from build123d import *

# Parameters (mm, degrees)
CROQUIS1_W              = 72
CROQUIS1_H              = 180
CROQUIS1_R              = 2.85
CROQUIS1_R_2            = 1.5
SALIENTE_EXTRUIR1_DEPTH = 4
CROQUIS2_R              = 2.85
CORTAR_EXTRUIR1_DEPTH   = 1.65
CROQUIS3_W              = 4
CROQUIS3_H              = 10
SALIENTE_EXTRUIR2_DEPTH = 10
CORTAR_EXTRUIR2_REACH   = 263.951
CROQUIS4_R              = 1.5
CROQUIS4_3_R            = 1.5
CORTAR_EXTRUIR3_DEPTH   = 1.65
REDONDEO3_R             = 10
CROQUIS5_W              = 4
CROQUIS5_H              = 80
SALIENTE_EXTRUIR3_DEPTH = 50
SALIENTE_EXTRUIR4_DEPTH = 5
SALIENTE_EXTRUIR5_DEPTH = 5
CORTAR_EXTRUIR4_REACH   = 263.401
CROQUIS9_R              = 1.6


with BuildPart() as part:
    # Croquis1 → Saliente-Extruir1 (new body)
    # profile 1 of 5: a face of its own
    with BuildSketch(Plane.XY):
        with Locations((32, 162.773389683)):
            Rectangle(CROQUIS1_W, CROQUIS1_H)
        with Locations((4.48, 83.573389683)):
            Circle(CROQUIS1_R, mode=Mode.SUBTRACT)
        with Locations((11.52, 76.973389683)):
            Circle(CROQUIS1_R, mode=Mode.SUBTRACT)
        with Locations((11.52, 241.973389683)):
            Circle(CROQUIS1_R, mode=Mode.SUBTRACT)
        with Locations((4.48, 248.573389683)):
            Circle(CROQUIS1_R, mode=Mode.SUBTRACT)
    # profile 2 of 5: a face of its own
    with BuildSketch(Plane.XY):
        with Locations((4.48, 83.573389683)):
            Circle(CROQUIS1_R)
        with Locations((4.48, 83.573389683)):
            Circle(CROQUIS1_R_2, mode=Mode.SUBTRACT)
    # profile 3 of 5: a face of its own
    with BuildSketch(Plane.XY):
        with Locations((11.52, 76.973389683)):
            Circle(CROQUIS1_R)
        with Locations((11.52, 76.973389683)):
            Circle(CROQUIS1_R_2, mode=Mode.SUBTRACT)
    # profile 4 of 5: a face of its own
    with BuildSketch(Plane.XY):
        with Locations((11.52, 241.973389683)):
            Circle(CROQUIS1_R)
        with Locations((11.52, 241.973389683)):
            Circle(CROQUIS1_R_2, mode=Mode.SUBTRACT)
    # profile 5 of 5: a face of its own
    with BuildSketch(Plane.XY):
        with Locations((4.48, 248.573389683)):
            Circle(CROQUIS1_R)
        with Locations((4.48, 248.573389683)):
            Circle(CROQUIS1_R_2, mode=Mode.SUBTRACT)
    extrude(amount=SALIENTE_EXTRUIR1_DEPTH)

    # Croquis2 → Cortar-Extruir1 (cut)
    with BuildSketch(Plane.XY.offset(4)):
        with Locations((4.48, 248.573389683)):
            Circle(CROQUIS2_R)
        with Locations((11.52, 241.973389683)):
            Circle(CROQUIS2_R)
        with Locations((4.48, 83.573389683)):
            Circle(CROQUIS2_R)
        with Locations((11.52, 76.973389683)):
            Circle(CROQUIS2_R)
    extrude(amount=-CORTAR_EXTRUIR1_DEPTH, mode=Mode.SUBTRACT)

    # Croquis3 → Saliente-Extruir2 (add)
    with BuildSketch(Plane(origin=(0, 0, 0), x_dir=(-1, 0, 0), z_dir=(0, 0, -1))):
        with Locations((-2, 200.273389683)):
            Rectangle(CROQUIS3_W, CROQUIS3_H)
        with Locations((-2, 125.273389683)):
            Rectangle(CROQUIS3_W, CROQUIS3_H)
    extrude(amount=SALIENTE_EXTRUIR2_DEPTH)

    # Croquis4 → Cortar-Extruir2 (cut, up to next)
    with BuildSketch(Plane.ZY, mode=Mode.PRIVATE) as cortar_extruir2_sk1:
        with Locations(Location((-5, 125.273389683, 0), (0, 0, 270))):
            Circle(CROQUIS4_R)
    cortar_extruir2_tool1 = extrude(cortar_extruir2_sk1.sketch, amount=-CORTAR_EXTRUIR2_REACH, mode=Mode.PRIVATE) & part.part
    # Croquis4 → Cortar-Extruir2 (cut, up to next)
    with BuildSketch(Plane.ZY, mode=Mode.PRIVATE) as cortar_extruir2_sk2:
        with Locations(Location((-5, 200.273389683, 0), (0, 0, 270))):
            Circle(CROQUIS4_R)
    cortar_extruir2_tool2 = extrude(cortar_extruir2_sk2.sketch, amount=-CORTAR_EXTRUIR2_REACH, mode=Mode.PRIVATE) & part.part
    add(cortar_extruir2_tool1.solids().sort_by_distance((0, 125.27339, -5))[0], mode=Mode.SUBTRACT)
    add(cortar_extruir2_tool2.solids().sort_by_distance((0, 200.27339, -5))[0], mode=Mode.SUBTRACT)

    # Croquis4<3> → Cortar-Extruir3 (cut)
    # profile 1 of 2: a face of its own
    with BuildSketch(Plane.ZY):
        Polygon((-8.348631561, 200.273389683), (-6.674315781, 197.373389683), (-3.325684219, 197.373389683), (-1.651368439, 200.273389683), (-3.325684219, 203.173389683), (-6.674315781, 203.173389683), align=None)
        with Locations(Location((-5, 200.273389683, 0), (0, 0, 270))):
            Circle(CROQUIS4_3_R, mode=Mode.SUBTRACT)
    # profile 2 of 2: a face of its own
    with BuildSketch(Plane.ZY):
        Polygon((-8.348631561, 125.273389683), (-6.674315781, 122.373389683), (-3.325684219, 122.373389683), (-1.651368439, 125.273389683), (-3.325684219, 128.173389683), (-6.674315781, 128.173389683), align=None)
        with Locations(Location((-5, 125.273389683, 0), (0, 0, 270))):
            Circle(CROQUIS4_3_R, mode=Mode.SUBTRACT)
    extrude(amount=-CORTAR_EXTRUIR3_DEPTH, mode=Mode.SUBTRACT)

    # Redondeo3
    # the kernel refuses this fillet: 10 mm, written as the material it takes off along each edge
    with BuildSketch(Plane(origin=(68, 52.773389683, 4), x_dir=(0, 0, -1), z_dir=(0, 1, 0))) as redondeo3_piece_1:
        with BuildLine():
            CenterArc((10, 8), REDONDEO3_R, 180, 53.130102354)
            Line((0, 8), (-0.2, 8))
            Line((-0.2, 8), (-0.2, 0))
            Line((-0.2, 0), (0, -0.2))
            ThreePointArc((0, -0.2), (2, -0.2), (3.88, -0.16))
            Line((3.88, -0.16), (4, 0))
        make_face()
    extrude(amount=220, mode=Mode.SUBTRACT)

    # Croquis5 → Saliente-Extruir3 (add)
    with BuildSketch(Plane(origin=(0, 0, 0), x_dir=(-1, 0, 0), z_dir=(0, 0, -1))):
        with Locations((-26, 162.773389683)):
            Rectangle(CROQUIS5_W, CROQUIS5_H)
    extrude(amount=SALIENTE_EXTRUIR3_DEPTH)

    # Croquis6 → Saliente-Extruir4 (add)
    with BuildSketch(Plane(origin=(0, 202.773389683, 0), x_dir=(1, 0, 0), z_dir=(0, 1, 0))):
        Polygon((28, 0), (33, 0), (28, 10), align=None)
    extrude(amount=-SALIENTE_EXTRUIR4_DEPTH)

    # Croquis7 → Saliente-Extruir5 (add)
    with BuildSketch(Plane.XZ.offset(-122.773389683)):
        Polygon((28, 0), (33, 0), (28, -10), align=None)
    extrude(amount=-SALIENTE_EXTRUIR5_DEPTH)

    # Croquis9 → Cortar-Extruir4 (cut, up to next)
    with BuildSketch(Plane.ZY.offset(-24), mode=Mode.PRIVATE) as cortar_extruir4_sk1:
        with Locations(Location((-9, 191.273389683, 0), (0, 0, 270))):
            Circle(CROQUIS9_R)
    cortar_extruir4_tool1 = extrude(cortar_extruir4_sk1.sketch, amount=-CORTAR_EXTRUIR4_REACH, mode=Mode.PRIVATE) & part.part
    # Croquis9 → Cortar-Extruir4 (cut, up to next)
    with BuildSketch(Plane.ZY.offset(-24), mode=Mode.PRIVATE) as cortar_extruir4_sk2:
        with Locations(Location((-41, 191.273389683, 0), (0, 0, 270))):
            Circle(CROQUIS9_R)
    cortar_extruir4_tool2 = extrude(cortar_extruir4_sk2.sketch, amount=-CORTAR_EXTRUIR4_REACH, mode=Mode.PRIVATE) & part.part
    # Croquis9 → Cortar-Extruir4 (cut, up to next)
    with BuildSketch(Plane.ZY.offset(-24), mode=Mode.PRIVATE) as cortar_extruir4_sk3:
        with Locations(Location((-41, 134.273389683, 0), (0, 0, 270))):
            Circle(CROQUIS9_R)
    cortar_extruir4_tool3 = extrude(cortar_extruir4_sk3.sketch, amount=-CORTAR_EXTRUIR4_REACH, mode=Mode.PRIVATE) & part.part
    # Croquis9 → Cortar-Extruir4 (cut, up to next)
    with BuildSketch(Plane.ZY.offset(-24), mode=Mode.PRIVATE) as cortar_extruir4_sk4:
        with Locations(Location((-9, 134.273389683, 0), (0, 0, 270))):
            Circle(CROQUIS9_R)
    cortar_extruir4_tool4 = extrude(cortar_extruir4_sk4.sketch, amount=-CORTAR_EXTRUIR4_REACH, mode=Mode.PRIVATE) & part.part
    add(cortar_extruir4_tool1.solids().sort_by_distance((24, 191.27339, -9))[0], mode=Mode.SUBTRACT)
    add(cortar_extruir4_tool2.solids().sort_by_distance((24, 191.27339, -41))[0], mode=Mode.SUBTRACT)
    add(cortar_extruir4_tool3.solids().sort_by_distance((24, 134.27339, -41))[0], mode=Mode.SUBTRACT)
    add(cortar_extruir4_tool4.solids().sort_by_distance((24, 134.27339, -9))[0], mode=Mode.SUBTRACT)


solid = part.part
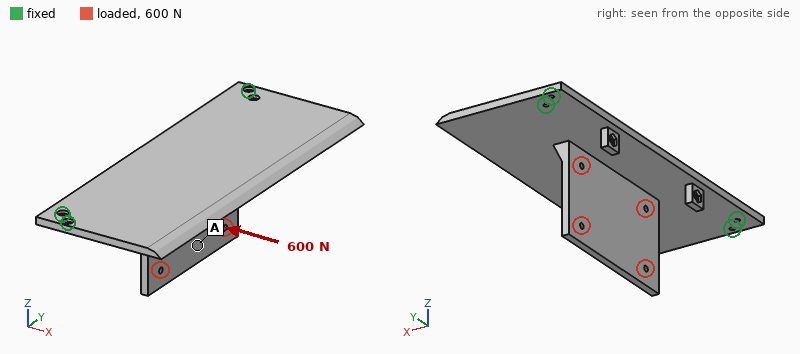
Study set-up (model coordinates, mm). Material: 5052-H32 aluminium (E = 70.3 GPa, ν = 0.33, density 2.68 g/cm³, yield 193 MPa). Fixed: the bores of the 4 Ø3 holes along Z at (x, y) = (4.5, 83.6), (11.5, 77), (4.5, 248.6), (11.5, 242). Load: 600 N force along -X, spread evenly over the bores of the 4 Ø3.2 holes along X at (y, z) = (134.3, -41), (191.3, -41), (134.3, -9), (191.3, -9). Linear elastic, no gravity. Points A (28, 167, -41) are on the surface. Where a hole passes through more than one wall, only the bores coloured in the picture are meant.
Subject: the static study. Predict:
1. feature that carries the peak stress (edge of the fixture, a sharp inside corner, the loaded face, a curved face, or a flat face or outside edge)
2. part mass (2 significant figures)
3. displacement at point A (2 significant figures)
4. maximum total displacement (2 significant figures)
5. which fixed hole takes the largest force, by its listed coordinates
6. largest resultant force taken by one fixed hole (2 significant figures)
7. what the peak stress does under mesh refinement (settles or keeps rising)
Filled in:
edge of the fixture
180 g
1.0 mm
1.3 mm
(11.5, 242)
780 N
keeps rising
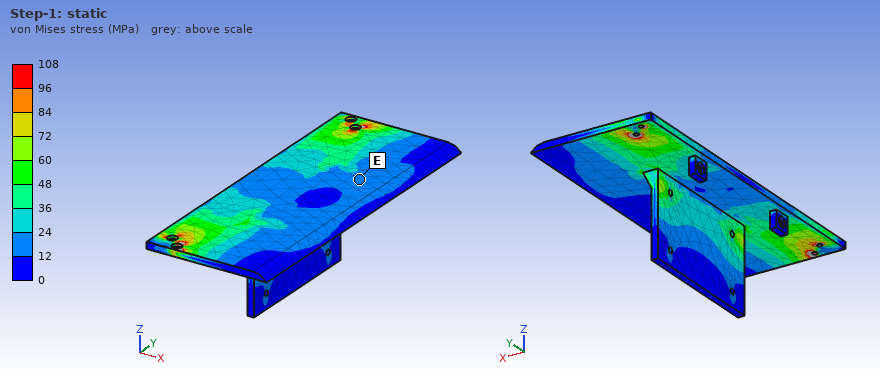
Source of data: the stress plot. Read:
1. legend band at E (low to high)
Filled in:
12 to 24 MPa
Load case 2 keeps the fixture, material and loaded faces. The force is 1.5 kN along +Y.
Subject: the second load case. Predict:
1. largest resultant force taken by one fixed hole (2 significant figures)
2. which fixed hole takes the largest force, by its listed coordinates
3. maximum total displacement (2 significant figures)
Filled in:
730 N
(11.5, 242)
0.31 mm
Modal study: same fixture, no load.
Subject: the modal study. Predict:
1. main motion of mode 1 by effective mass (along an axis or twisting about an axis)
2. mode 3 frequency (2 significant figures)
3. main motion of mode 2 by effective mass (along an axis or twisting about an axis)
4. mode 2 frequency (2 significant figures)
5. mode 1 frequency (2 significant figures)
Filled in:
along Z
1000 Hz
along Z
800 Hz
420 Hz
